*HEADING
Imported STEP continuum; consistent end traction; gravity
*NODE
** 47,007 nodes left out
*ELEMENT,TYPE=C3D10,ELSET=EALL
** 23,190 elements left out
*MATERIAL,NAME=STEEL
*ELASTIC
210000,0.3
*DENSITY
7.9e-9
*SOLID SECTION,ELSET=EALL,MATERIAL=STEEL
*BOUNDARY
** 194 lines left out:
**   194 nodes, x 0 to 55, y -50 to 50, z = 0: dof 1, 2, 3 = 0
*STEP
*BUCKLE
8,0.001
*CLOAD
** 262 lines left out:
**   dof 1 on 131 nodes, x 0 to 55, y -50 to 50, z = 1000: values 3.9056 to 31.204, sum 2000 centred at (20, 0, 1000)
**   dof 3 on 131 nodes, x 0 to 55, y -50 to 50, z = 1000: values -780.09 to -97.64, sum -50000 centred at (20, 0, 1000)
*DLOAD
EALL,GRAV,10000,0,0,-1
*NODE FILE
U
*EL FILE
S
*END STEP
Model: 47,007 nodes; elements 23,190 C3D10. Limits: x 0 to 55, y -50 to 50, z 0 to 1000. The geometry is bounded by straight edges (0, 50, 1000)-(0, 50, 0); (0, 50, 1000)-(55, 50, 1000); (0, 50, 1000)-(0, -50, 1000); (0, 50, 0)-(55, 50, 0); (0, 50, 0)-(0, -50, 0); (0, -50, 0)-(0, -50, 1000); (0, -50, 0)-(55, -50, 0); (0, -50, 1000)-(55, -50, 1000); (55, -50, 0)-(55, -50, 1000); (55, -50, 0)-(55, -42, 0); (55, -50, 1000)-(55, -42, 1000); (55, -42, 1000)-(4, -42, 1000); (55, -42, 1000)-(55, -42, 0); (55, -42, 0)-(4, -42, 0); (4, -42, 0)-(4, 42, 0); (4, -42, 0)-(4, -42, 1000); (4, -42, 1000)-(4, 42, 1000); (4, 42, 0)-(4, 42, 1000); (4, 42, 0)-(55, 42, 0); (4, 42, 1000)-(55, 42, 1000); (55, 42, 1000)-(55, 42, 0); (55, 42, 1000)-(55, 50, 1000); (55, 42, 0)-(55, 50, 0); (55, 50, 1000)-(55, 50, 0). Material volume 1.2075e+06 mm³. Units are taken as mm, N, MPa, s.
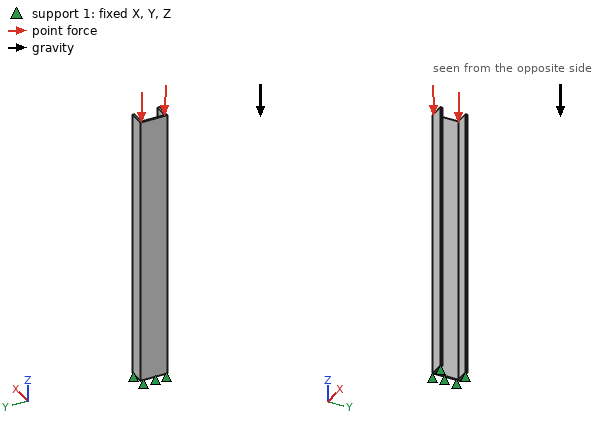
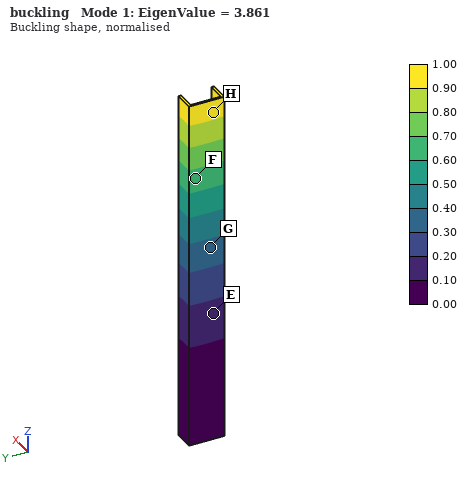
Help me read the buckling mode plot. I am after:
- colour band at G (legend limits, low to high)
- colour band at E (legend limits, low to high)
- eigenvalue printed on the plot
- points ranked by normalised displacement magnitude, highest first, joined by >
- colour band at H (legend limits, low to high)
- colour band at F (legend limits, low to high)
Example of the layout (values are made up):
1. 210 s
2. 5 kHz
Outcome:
1. 0.30 to 0.40
2. 0.10 to 0.20
3. 3.861
4. H > F > G > E
5. 0.90 to 1.00
6. 0.60 to 0.70
